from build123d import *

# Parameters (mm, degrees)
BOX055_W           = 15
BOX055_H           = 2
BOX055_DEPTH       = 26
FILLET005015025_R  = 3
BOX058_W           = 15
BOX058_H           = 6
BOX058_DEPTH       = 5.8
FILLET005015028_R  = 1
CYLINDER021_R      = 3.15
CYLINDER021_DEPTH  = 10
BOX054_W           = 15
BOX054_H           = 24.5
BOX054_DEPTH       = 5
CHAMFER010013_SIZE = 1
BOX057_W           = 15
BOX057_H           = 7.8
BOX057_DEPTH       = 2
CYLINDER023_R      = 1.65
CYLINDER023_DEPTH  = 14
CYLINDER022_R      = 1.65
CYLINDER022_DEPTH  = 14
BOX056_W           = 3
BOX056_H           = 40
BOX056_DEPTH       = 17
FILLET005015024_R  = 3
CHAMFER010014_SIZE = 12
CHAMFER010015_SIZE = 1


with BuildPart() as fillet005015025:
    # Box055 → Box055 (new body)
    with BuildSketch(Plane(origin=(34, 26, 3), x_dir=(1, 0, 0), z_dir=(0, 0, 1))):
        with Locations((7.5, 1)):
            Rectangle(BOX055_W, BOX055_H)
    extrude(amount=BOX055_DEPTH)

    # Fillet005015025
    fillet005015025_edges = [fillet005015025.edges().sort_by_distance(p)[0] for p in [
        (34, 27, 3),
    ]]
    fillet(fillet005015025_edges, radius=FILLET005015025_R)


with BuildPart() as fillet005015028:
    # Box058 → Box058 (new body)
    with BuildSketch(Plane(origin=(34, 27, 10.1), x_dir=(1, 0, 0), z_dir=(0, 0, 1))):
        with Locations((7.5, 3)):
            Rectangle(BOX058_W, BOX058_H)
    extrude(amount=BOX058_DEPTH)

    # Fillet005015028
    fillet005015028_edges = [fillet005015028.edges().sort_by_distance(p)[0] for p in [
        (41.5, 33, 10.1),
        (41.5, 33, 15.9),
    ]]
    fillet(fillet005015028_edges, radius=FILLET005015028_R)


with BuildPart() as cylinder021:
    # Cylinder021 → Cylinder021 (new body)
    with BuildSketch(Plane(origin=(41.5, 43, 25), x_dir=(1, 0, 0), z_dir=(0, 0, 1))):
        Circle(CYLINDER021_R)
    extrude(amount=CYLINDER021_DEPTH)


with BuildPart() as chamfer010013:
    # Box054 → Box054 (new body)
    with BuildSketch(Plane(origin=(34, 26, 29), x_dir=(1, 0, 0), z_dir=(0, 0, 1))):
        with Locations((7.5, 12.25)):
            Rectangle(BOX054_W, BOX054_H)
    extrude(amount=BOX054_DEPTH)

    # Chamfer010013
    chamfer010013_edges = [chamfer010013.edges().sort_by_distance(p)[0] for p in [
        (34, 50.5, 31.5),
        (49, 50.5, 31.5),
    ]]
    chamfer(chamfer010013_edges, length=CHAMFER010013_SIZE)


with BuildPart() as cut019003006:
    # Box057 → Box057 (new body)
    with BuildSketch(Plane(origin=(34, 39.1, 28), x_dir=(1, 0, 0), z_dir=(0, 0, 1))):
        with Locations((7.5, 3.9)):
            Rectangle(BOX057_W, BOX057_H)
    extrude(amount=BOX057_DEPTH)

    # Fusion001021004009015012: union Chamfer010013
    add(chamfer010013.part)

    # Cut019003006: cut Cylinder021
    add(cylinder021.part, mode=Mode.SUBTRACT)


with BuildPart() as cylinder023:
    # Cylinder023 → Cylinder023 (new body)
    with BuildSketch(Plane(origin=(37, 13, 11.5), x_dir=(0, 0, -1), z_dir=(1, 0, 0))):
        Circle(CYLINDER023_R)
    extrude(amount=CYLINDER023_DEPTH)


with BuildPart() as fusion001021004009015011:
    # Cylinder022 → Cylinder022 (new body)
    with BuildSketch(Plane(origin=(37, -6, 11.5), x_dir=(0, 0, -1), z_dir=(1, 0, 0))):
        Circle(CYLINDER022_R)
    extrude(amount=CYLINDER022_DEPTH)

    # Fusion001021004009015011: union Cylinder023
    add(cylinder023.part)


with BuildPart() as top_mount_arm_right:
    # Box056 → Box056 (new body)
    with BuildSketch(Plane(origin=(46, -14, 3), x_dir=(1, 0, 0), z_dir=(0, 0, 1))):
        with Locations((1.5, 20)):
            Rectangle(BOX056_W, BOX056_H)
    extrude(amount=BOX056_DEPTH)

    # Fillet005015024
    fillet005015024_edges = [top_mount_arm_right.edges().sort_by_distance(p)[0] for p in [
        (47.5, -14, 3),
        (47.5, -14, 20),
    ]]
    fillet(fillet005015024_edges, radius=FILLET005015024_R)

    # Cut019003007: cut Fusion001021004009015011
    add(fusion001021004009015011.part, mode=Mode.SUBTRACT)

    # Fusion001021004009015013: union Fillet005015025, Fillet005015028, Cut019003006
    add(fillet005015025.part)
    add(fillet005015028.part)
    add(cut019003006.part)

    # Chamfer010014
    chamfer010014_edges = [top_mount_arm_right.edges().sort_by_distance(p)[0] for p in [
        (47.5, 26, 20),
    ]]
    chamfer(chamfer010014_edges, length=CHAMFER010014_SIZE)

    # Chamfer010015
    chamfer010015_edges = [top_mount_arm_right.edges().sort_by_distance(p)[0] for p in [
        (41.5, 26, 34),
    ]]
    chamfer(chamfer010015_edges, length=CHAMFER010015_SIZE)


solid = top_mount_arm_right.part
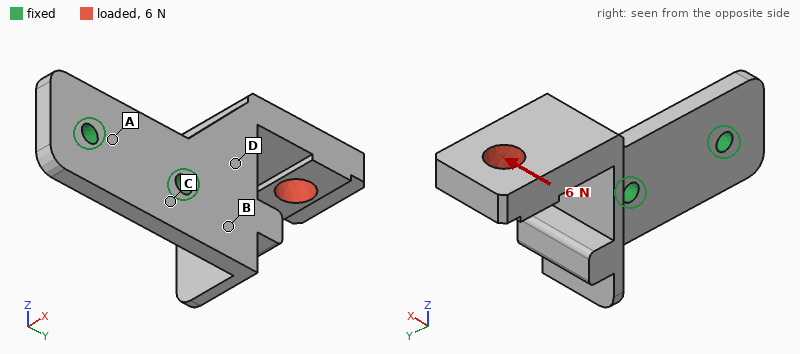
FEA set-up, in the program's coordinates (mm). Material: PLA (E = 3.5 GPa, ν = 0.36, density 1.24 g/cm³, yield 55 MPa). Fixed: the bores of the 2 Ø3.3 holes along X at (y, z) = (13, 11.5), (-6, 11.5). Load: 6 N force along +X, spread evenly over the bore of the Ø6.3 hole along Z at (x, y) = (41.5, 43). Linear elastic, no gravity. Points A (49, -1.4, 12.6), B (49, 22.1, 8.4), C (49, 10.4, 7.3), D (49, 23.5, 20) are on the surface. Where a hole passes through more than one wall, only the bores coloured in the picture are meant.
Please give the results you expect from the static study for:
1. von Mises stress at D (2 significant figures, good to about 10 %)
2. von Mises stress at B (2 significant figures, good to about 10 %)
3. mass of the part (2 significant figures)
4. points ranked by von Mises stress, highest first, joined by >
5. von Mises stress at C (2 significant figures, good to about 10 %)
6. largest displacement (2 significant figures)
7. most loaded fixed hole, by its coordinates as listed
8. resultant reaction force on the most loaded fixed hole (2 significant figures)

3.9 MPa
5.1 MPa
6.4 g
B > D > C > A
1.6 MPa
0.84 mm
(13, 11.5)
8.1 N
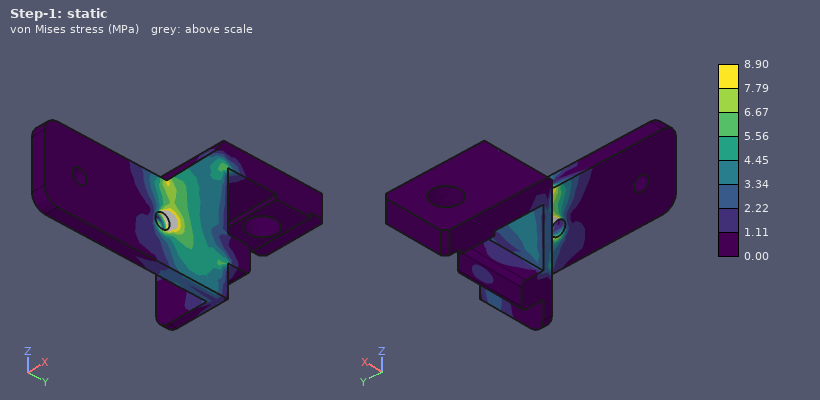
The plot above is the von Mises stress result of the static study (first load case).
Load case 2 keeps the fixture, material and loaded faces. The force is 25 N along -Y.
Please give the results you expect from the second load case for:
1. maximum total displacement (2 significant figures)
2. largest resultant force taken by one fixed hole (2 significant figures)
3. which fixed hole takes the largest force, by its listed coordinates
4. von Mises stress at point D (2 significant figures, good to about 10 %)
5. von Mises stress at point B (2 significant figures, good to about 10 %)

0.85 mm
27 N
(13, 11.5)
4.5 MPa
4.7 MPa
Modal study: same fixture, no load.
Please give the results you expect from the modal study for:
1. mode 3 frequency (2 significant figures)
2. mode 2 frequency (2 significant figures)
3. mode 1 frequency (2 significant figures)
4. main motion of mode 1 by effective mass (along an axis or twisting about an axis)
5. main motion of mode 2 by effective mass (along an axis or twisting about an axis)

1300 Hz
750 Hz
360 Hz
along X
along Z
